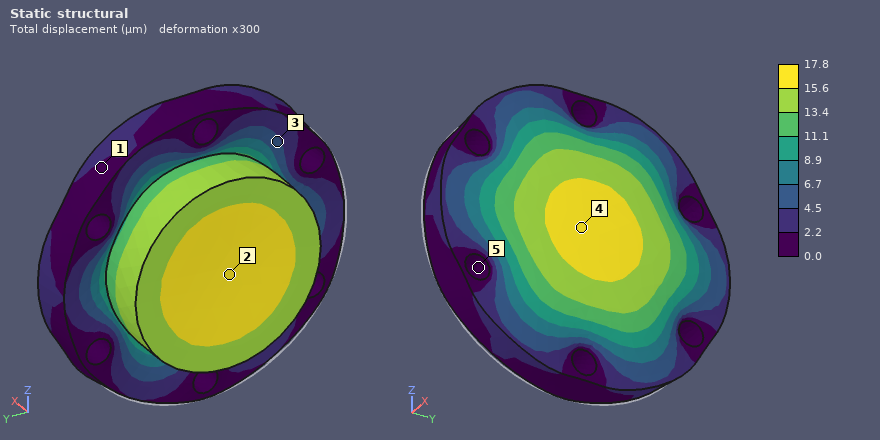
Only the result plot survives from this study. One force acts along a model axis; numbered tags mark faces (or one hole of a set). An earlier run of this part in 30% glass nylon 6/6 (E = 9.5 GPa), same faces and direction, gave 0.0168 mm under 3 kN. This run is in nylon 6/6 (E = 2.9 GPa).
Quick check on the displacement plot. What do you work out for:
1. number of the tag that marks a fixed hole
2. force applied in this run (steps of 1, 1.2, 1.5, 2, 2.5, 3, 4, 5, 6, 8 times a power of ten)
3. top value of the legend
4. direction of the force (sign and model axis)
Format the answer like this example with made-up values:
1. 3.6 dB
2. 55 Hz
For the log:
1. 5
2. 1 kN
3. 17.8 µm
4. +X
